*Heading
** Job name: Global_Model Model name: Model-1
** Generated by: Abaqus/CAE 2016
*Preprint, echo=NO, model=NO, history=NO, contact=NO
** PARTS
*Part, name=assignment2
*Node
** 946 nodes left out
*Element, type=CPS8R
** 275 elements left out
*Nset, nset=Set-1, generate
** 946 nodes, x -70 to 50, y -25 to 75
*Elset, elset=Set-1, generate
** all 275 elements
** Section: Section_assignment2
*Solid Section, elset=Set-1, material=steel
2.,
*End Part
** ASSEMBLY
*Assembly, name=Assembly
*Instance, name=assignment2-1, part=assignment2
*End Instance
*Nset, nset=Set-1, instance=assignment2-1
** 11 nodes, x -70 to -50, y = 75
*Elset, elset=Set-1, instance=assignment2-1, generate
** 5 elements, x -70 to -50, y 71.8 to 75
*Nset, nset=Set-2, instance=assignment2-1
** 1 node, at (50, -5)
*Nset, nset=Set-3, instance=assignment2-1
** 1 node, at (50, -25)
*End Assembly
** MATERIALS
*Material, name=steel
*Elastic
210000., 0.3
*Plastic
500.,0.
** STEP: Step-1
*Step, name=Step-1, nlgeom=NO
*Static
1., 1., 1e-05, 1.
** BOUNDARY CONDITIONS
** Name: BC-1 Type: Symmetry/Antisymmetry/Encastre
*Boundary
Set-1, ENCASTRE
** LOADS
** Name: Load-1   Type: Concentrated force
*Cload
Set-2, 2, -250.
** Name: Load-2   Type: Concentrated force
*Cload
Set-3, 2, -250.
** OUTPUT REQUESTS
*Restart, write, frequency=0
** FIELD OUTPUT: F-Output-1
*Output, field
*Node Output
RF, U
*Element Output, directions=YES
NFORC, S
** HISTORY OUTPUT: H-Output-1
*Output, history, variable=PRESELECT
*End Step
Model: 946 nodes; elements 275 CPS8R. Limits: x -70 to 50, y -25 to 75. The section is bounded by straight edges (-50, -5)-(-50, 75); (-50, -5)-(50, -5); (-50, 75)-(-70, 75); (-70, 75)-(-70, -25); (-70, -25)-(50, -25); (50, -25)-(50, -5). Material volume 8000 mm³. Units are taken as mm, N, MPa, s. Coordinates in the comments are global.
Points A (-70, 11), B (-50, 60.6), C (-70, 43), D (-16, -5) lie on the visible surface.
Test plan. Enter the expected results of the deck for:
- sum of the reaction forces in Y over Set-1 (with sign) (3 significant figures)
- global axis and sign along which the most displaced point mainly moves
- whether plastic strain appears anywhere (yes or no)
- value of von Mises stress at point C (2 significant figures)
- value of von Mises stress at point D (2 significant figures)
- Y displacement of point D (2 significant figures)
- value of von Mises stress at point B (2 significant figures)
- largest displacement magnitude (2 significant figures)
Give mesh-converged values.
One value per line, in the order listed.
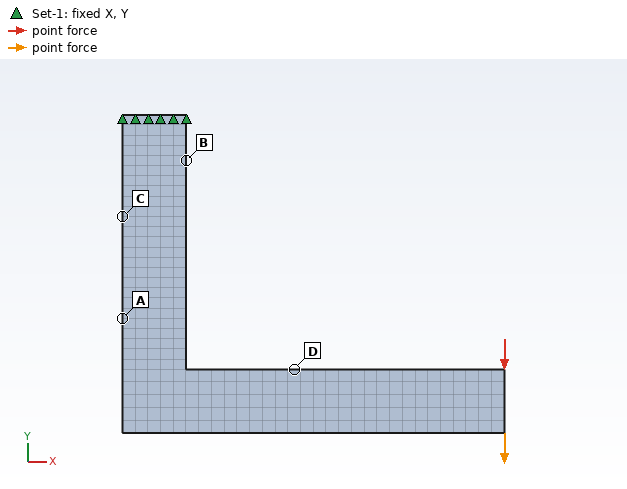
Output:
500 N
-Y
yes
400 MPa
250 MPa
-0.91 mm
420 MPa
2.9 mm
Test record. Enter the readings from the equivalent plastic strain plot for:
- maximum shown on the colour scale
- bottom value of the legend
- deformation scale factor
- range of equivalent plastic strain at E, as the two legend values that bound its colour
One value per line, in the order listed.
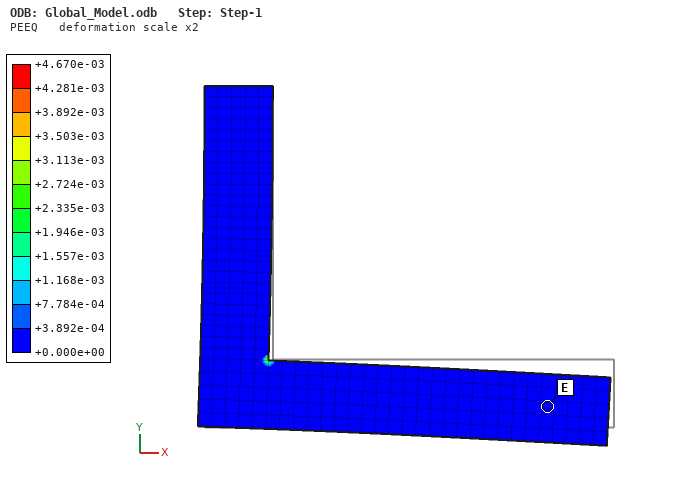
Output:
+4.670e-03
+0.000e+00
2
+0.000e+00 to +3.892e-04
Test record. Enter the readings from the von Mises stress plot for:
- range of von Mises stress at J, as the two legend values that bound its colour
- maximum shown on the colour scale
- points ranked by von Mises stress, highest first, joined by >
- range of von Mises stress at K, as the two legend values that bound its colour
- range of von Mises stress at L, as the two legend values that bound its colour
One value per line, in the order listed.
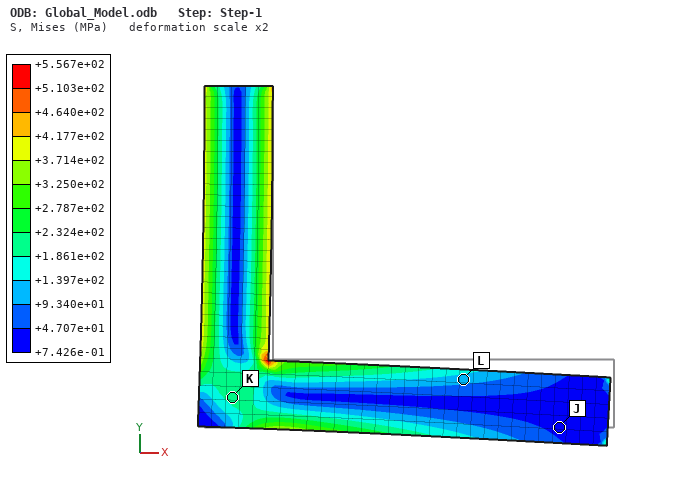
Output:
+7.426e-01 to +4.707e+01 MPa
+5.567e+02 MPa
K > L > J
+1.861e+02 to +2.324e+02 MPa
+9.340e+01 to +1.397e+02 MPa
